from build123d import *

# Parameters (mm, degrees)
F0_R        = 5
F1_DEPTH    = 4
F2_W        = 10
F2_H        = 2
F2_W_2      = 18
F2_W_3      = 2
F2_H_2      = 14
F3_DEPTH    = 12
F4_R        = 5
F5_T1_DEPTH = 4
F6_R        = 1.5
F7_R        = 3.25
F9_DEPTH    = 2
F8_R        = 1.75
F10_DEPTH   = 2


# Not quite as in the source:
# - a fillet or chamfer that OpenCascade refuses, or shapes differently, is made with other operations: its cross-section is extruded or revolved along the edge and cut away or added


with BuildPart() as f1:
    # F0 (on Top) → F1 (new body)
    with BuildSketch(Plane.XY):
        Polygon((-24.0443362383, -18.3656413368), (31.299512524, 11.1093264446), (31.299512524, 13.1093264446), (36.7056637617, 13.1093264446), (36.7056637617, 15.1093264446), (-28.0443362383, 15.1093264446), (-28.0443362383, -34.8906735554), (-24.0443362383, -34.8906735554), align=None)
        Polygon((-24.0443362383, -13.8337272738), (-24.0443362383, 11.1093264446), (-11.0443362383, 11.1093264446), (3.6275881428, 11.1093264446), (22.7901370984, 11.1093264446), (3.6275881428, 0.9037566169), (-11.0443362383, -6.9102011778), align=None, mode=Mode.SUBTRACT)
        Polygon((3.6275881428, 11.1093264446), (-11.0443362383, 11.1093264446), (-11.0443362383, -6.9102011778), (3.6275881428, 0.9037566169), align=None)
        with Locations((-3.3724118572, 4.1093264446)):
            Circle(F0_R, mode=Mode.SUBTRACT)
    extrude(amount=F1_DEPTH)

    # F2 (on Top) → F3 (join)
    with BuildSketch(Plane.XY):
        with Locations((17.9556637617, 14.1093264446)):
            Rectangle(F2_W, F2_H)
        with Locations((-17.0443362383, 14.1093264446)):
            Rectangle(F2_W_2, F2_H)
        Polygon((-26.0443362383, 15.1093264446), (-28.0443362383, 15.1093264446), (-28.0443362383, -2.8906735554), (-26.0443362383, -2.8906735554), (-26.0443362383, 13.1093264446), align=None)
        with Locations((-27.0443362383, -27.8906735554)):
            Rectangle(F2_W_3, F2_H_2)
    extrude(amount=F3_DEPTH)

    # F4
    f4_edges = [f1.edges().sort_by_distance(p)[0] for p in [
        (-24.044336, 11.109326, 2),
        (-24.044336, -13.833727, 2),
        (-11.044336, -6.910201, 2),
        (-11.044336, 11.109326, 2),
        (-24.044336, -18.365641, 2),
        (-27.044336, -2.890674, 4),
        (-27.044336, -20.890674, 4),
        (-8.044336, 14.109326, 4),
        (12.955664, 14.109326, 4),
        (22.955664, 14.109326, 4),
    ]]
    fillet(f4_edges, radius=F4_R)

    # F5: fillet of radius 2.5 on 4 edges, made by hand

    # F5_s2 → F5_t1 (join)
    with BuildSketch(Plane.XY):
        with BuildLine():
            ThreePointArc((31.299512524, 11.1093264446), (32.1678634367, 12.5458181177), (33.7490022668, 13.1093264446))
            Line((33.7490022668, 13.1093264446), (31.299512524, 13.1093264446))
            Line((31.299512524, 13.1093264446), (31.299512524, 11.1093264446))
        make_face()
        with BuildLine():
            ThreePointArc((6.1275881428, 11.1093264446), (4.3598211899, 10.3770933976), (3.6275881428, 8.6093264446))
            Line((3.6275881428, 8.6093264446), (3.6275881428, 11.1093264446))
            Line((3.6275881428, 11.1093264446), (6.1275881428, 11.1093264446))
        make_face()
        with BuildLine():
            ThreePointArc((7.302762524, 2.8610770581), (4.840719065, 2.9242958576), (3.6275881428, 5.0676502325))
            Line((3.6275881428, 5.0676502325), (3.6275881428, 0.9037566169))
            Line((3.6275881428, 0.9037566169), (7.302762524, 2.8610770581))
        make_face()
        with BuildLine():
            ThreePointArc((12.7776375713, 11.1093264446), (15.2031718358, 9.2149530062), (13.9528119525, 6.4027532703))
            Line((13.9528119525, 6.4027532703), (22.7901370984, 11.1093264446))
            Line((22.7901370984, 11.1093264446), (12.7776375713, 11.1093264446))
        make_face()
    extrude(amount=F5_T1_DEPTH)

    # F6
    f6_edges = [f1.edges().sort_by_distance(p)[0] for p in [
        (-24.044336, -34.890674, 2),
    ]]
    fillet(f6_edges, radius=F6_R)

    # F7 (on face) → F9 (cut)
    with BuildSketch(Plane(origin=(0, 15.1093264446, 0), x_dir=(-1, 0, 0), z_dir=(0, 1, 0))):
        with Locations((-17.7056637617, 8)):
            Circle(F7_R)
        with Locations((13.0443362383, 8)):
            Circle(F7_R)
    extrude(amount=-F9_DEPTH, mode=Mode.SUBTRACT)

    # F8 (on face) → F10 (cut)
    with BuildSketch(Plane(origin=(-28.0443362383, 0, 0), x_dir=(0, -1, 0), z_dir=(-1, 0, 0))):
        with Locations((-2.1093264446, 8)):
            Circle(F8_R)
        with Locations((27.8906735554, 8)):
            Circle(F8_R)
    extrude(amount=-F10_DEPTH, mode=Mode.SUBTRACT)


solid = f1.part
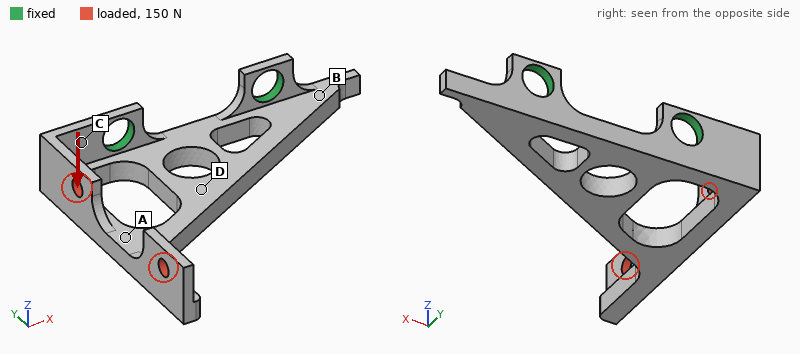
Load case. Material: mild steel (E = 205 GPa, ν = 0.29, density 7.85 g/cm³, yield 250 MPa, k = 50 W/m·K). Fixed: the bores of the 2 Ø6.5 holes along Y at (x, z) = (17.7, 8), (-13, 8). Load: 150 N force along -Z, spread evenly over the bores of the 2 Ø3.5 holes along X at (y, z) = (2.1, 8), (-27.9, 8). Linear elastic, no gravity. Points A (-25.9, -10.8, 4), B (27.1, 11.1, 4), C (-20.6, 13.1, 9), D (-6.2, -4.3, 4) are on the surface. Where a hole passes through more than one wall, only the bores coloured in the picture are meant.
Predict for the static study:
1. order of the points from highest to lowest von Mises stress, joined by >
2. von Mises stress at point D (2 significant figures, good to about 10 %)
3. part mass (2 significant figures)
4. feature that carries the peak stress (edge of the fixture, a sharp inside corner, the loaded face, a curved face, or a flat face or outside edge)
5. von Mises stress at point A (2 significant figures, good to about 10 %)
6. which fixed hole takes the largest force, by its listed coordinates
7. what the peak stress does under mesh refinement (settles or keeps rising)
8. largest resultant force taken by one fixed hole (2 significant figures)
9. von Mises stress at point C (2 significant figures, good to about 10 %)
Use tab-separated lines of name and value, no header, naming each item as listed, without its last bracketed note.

order of the points from highest to lowest von Mises stress, joined by >	C > A > D > B
von Mises stress at point D	47 MPa
part mass	33 g
feature that carries the peak stress	edge of the fixture
von Mises stress at point A	62 MPa
which fixed hole takes the largest force, by its listed coordinates	(-13, 8)
what the peak stress does under mesh refinement	keeps rising
largest resultant force taken by one fixed hole	160 N
von Mises stress at point C	140 MPa
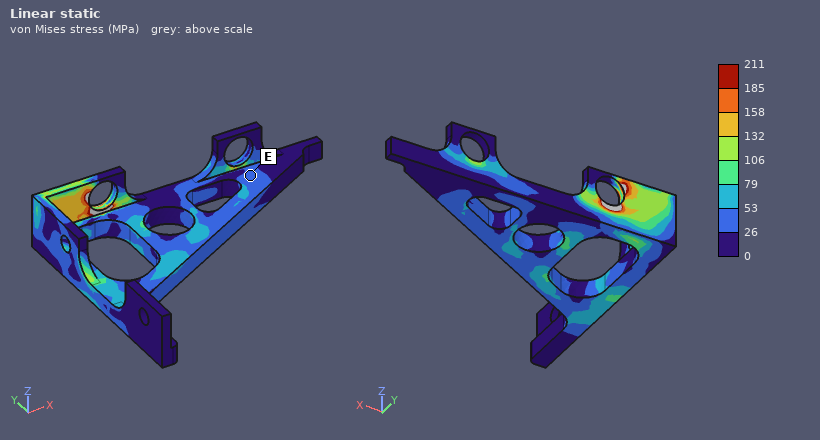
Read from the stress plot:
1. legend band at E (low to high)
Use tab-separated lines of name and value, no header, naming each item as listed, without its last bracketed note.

legend band at E	26 to 53 MPa
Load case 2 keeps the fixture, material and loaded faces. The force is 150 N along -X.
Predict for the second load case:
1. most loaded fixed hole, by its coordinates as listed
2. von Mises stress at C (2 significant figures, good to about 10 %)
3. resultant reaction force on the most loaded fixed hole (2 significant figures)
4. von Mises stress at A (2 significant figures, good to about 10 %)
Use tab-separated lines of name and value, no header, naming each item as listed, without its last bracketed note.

most loaded fixed hole, by its coordinates as listed	(17.7, 8)
von Mises stress at C	27 MPa
resultant reaction force on the most loaded fixed hole	150 N
von Mises stress at A	19 MPa
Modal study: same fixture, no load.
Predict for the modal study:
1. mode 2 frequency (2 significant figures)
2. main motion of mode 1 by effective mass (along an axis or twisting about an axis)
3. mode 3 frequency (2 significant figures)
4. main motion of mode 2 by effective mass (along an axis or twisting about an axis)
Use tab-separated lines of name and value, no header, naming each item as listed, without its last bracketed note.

mode 2 frequency	4200 Hz
main motion of mode 1 by effective mass	along Z
mode 3 frequency	4800 Hz
main motion of mode 2 by effective mass	along X
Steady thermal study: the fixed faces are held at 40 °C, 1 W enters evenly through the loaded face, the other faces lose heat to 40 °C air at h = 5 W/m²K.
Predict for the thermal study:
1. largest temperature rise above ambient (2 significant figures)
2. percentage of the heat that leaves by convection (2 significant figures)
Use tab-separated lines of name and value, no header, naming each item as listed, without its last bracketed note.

largest temperature rise above ambient	17 K
percentage of the heat that leaves by convection	9.8 %
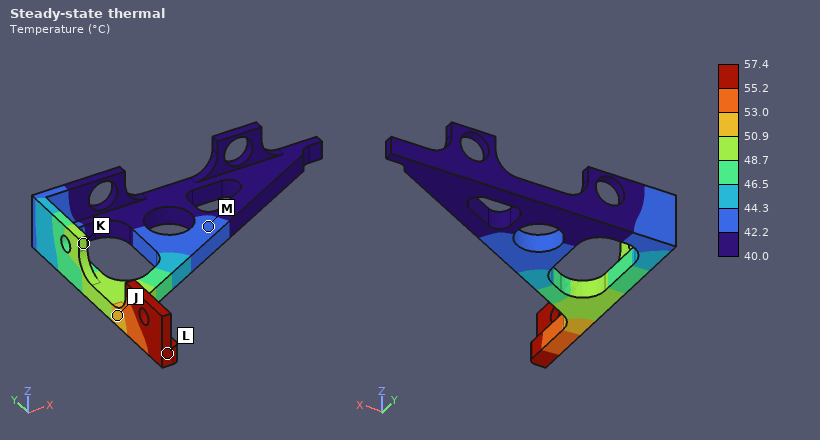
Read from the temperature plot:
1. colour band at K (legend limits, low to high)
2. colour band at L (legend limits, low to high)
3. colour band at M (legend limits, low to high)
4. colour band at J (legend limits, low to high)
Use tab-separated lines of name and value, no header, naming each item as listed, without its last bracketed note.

colour band at K	48.7 to 50.9 °C
colour band at L	55.2 to 57.4 °C
colour band at M	42.2 to 44.3 °C
colour band at J	50.9 to 53.0 °C
